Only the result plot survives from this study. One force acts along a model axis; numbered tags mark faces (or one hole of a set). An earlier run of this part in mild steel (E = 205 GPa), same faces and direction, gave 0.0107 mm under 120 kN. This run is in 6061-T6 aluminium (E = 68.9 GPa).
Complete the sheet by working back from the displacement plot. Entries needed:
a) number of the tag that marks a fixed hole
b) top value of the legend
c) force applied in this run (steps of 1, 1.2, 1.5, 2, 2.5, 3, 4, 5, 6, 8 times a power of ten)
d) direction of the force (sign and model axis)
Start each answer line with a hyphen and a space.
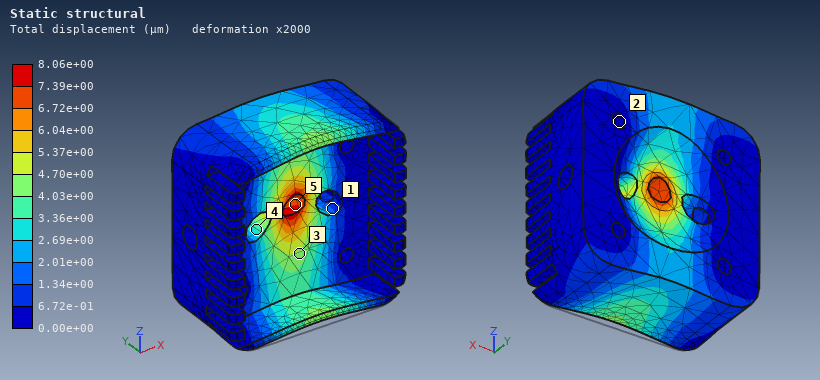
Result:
- 2
- 8.06e+00 µm
- 30 kN
- +Z
